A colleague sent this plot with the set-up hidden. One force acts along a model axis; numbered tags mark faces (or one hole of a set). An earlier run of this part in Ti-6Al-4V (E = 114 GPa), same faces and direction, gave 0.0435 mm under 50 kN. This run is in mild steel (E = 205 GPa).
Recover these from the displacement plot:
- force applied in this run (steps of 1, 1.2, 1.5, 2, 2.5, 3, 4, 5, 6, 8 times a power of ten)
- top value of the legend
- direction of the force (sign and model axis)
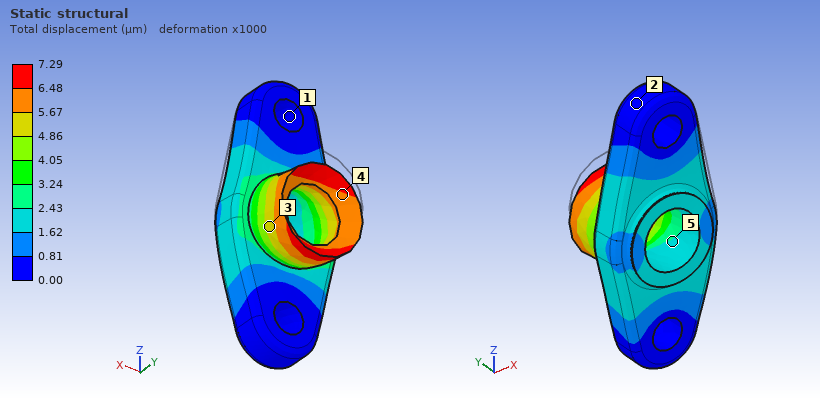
15 kN
7.29 µm
-Z
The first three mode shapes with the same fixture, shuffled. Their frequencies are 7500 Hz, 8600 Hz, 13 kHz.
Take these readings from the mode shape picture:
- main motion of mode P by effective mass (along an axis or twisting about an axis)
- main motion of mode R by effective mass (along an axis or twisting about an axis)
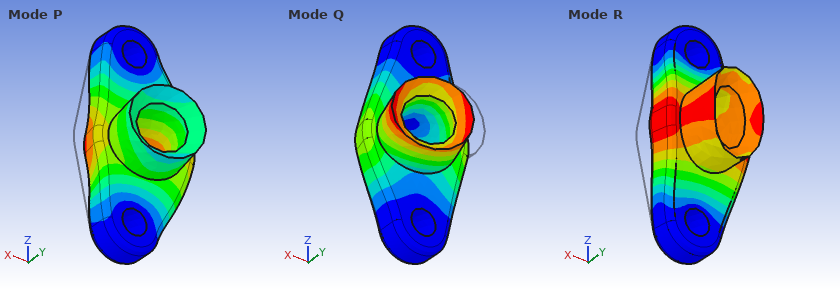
along X
along Y
